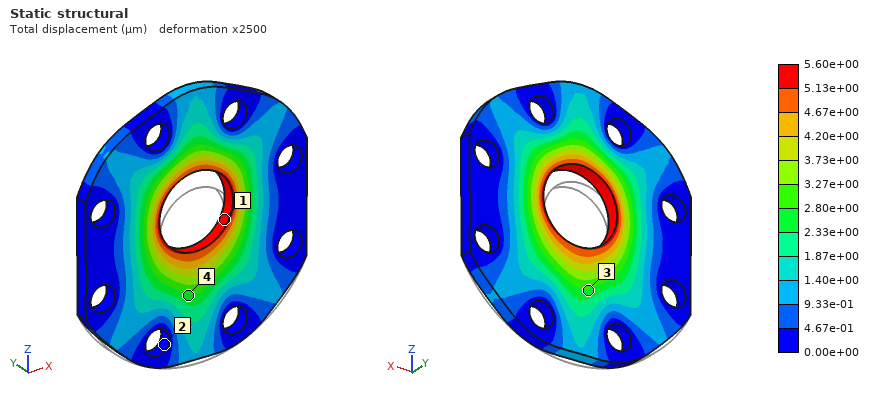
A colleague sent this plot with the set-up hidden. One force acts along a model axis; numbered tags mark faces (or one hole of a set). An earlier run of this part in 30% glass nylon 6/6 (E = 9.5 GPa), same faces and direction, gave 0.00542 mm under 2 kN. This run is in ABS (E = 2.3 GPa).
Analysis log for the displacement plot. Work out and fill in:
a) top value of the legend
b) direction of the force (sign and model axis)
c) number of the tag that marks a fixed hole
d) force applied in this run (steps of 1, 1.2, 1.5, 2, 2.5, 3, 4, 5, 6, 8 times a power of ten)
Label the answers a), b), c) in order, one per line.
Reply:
a) 5.60e+00 µm
b) +Z
c) 2
d) 500 N
